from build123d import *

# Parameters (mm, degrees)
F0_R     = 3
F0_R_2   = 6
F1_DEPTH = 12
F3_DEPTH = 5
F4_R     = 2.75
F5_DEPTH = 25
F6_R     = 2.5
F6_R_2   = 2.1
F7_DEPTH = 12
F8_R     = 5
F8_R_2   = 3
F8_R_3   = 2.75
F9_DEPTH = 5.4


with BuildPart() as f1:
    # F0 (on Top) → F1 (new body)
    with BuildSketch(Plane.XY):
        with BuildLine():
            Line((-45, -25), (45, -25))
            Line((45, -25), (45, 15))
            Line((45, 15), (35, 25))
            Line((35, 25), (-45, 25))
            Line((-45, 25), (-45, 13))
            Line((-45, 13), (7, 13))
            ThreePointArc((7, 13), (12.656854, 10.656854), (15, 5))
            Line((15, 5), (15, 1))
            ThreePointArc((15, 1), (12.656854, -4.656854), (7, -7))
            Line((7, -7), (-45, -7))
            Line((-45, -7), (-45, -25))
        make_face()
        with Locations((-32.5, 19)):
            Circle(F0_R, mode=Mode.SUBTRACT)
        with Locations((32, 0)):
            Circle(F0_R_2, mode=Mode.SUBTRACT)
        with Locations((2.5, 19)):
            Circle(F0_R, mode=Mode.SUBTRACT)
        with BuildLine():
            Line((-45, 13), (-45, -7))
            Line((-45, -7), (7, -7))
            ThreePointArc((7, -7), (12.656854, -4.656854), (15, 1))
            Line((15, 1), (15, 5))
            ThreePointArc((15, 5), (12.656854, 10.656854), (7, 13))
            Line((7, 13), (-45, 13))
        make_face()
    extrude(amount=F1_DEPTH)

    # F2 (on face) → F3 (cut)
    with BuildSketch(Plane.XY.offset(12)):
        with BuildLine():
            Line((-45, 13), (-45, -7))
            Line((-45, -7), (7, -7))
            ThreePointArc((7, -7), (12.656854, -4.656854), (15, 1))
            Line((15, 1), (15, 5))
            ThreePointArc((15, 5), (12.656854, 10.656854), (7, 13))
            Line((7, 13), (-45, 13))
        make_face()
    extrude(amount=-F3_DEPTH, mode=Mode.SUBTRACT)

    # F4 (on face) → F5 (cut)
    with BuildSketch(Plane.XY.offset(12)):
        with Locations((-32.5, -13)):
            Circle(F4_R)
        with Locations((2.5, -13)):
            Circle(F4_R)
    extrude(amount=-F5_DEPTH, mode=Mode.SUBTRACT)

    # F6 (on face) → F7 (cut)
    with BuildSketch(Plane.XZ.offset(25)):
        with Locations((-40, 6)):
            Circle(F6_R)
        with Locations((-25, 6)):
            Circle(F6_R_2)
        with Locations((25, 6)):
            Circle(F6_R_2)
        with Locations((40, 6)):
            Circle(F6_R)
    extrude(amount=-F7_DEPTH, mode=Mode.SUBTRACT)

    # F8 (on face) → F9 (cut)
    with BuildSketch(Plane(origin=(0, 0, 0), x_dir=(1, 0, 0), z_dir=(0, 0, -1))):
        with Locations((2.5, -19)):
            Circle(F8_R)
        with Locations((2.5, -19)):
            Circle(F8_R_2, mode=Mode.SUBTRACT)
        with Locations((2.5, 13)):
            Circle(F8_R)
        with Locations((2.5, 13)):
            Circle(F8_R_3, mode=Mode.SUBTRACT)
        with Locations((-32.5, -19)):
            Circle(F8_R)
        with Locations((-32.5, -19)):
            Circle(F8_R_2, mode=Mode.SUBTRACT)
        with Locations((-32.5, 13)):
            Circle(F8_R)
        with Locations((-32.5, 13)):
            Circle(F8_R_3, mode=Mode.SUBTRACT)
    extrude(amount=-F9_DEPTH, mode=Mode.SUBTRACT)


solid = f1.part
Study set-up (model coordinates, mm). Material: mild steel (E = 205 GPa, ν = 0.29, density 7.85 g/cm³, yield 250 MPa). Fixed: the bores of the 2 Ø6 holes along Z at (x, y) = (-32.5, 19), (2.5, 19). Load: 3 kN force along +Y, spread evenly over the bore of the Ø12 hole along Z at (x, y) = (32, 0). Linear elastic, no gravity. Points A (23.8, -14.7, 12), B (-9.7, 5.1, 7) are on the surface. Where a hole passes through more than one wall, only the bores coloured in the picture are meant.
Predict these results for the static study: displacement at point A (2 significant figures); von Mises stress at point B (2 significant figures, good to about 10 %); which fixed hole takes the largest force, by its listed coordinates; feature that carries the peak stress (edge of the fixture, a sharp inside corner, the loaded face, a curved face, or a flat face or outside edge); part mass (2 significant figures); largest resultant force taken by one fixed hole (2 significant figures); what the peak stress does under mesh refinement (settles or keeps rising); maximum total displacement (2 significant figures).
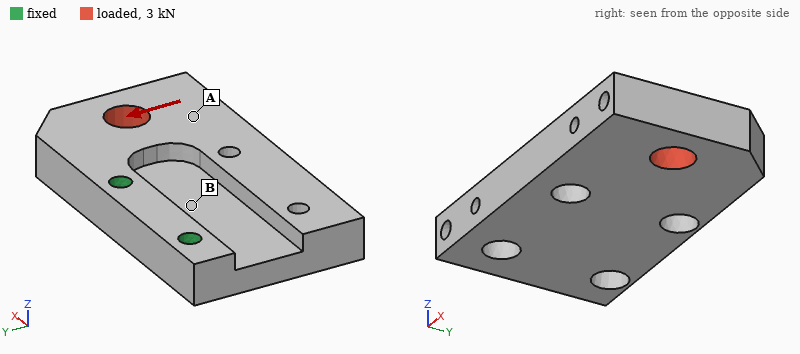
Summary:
20 µm
26 MPa
(2.5, 19)
edge of the fixture
340 g
5.0 kN
keeps rising
31 µm
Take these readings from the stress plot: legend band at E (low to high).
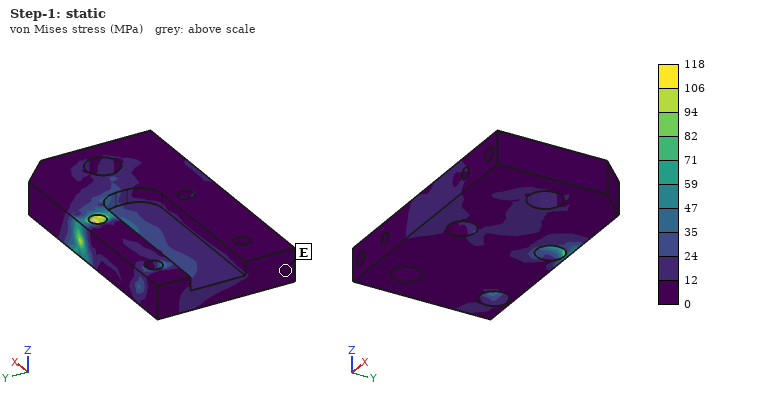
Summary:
0 to 12 MPa
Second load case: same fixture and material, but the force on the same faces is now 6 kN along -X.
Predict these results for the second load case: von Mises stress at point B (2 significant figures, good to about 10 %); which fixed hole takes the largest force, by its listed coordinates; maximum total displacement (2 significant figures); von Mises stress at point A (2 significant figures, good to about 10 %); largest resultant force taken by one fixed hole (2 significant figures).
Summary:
32 MPa
(2.5, 19)
25 µm
10 MPa
4.8 kN
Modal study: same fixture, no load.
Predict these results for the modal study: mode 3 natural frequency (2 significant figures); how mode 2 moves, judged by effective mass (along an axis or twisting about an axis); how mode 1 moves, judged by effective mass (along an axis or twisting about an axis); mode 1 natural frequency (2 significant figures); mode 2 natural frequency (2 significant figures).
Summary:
5100 Hz
twisting about Y
along Z
1800 Hz
3100 Hz
